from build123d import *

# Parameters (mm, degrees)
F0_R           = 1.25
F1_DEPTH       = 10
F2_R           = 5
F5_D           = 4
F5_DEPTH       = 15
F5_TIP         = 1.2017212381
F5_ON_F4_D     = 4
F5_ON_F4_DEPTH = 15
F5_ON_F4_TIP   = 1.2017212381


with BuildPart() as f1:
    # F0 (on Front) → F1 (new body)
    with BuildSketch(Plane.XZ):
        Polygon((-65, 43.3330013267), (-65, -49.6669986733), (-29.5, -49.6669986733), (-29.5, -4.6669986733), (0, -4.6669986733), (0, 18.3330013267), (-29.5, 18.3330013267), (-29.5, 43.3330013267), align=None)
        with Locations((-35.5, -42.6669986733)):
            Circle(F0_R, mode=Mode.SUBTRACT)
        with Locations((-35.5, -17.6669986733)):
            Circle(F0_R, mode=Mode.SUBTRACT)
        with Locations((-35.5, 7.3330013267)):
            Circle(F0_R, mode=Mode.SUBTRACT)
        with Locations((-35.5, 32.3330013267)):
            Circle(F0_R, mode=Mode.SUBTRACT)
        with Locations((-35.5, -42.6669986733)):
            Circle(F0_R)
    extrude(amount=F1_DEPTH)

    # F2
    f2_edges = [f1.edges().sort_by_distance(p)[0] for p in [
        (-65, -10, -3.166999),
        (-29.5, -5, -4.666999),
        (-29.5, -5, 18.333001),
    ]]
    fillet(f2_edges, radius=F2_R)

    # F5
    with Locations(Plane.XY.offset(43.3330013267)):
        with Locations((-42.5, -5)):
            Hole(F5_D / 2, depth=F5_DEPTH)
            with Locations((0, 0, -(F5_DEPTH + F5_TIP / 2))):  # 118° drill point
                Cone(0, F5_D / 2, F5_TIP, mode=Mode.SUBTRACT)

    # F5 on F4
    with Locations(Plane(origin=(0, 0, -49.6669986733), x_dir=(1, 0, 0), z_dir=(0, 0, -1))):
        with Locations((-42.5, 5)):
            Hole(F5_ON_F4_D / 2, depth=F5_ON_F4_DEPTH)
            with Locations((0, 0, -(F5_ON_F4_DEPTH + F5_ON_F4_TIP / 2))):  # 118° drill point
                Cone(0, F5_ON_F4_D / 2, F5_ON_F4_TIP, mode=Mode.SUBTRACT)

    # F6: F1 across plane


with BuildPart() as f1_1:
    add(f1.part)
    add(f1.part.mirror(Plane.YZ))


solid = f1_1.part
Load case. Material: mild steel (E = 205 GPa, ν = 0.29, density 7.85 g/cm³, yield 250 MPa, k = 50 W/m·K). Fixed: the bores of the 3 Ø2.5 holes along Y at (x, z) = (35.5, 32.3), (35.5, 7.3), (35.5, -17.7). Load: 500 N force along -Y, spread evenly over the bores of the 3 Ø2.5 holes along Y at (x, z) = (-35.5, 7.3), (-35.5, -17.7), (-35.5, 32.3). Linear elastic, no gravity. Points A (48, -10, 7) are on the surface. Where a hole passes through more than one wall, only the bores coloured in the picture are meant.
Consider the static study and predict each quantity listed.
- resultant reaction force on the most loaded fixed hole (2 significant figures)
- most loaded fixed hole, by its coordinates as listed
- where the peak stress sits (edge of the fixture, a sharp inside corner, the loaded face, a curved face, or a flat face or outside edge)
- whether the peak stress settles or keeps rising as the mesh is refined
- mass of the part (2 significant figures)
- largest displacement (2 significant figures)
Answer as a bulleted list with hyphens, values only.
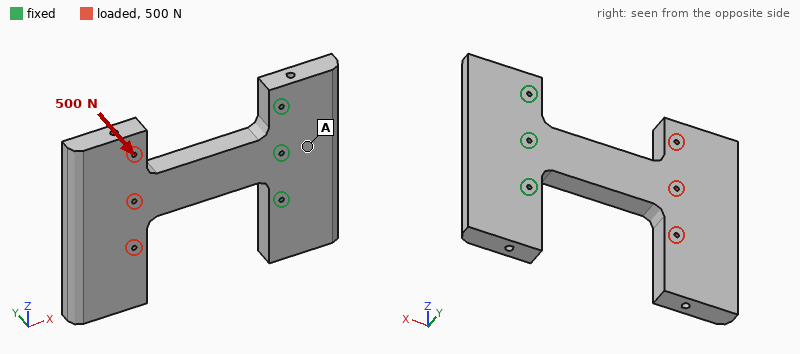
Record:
- 800 N
- (35.5, 7.3)
- edge of the fixture
- keeps rising
- 610 g
- 0.26 mm
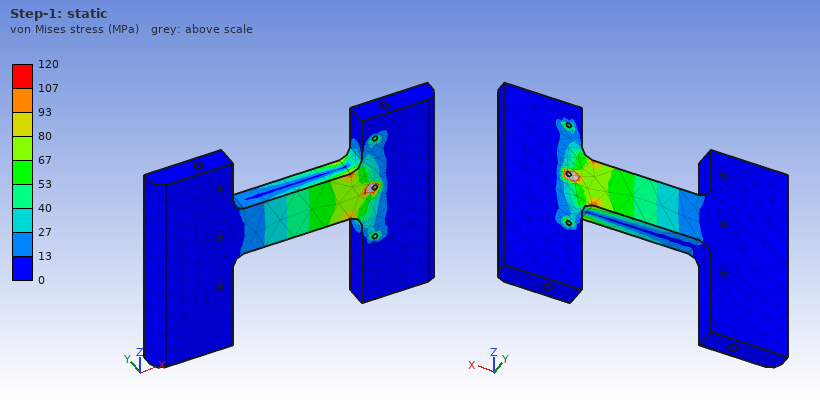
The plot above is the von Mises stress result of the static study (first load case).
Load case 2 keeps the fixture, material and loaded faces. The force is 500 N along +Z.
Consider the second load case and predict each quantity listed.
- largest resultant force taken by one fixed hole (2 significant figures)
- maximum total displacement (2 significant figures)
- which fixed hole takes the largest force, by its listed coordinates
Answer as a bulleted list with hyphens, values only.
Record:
- 780 N
- 59 µm
- (35.5, -17.7)
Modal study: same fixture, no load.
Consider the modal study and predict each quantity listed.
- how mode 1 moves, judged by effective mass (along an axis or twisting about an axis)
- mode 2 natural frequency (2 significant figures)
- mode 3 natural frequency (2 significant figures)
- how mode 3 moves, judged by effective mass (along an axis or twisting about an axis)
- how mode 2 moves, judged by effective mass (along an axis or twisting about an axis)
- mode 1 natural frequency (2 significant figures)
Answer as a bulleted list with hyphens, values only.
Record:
- along Y
- 900 Hz
- 950 Hz
- twisting about X
- along Z
- 420 Hz
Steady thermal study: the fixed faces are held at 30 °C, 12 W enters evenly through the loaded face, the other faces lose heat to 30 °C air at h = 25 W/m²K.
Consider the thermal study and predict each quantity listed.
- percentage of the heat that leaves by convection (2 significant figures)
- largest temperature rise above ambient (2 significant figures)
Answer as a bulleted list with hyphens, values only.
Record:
- 66 %
- 34 K
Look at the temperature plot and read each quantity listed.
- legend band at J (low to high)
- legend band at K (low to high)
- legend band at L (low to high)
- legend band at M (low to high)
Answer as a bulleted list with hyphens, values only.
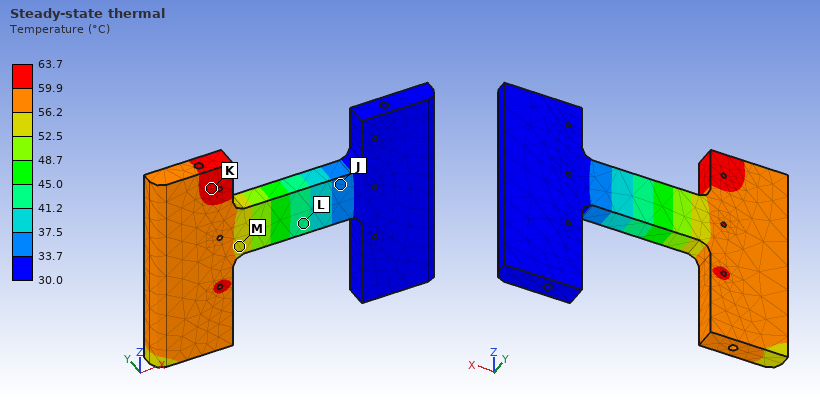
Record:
- 33.7 to 37.5 °C
- 59.9 to 63.7 °C
- 41.2 to 45.0 °C
- 52.5 to 56.2 °C
